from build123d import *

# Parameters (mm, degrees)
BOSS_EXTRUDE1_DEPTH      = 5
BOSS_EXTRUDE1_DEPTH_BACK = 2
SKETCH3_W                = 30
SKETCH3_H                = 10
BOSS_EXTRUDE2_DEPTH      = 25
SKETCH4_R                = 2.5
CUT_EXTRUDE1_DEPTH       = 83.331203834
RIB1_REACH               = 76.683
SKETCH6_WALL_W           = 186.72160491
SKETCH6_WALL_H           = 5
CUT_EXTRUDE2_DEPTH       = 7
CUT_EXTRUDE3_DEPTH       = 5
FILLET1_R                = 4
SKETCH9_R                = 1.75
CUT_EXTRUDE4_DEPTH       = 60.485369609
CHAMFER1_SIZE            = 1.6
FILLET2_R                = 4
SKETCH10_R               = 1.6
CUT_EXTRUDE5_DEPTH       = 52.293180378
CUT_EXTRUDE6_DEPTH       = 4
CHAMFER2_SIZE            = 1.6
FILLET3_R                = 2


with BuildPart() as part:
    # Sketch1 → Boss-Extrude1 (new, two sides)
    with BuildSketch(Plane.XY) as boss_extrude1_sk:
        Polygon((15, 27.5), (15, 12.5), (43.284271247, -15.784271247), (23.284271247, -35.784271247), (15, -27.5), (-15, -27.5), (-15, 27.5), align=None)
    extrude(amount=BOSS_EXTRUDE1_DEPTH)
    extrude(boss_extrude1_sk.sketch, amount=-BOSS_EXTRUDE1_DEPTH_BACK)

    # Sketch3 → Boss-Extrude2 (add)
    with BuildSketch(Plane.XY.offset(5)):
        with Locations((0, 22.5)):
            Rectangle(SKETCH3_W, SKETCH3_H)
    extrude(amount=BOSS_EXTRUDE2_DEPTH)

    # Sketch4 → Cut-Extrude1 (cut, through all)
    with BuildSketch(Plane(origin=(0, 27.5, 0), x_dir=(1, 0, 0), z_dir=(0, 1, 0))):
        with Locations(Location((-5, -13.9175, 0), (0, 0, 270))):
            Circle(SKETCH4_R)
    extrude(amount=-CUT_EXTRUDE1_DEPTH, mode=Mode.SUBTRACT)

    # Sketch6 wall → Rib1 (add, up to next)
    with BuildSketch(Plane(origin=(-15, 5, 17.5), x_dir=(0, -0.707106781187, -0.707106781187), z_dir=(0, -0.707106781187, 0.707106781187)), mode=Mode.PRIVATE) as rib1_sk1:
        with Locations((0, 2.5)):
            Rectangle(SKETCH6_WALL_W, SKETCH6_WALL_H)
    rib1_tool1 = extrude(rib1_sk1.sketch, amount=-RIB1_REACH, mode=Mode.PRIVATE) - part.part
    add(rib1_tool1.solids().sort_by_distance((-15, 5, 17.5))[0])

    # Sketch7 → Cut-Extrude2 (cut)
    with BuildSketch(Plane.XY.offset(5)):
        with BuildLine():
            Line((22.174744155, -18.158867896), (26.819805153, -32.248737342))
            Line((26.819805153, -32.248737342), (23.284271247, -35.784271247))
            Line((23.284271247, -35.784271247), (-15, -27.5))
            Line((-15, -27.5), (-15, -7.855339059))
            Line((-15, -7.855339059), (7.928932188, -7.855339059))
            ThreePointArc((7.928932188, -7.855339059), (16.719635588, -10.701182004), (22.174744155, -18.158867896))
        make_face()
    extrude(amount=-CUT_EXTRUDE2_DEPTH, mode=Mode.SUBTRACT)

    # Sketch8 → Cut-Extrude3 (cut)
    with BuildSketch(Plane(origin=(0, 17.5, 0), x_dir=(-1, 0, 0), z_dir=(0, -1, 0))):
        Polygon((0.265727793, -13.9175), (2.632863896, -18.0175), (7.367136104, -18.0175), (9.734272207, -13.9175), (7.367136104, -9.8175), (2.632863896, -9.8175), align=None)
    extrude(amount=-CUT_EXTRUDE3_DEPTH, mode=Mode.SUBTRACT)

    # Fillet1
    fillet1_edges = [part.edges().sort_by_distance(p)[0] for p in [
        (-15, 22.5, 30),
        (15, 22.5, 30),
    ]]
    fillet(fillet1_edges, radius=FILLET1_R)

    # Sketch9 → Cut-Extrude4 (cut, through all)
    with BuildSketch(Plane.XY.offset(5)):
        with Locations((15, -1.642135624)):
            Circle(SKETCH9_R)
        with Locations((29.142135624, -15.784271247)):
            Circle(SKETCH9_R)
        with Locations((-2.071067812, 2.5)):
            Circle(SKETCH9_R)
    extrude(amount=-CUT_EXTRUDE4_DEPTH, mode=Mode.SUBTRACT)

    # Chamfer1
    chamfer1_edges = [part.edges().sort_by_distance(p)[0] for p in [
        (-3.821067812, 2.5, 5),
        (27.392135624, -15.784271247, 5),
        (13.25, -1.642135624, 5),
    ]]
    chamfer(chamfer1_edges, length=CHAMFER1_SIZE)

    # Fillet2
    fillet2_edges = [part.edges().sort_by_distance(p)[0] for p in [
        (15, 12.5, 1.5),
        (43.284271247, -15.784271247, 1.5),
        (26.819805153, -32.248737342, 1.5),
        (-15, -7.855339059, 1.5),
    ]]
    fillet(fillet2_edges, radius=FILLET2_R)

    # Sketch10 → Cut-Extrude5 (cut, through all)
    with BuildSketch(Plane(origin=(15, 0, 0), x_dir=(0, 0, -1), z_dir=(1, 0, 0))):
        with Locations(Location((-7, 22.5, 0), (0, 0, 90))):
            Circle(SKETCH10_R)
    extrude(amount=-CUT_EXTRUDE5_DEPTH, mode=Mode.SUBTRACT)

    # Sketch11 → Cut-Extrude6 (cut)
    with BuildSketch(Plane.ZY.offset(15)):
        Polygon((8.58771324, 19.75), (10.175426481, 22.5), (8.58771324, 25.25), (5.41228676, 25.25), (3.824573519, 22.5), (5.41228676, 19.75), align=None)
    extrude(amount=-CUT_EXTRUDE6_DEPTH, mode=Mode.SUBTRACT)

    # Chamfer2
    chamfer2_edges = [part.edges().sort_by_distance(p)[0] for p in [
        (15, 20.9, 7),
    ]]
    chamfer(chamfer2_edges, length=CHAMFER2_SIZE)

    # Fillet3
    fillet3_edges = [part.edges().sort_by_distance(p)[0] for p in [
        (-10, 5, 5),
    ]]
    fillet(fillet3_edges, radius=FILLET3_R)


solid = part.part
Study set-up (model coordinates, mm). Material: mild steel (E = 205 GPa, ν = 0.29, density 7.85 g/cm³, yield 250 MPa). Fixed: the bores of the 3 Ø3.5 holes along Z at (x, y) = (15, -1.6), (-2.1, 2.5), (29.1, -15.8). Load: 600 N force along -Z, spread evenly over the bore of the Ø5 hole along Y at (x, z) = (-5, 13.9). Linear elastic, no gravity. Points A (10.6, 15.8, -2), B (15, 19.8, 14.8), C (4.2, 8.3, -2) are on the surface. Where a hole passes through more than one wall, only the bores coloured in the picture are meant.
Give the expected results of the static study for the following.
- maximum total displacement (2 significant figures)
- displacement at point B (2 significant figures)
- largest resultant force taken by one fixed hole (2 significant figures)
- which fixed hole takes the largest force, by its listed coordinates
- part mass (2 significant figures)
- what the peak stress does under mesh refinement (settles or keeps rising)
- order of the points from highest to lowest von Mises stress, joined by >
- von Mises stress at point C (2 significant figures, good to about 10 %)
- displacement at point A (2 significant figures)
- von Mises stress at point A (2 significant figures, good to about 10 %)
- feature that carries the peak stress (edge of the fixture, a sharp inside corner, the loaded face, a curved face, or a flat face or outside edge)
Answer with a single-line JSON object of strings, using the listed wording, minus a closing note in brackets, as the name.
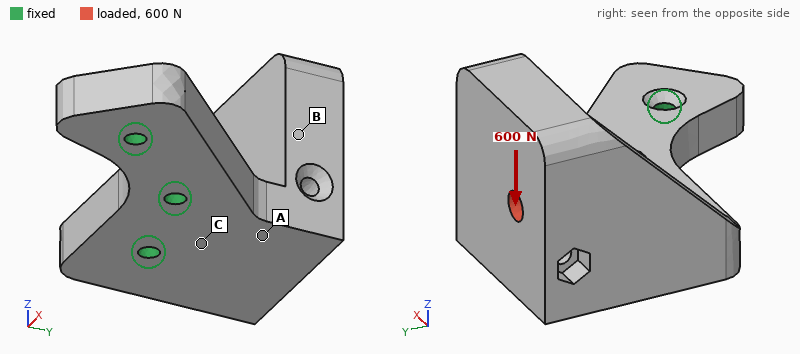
{"maximum total displacement": "30 µm", "displacement at point B": "14 µm", "largest resultant force taken by one fixed hole": "700 N", "which fixed hole takes the largest force, by its listed coordinates": "(-2.1, 2.5)", "part mass": "150 g", "what the peak stress does under mesh refinement": "keeps rising", "order of the points from highest to lowest von Mises stress, joined by >": "C > A > B", "von Mises stress at point C": "28 MPa", "displacement at point A": "7.1 µm", "von Mises stress at point A": "18 MPa", "feature that carries the peak stress": "edge of the fixture"}
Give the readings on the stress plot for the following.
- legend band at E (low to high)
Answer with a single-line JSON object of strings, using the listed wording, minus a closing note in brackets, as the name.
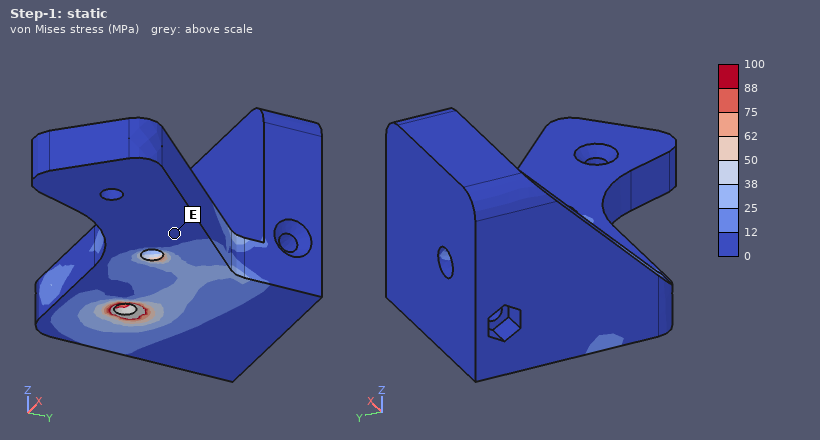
{"legend band at E": "0 to 12 MPa"}
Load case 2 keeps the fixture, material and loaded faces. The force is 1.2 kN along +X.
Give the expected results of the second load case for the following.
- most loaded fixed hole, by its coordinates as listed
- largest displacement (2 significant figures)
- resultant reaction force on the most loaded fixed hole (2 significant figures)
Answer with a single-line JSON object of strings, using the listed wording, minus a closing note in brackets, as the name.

{"most loaded fixed hole, by its coordinates as listed": "(-2.1, 2.5)", "largest displacement": "24 µm", "resultant reaction force on the most loaded fixed hole": "1.7 kN"}
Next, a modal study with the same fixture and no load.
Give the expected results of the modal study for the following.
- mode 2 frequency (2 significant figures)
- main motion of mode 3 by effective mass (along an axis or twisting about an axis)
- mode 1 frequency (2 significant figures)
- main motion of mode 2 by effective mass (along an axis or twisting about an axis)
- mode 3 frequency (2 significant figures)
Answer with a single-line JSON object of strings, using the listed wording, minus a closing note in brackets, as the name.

{"mode 2 frequency": "4500 Hz", "main motion of mode 3 by effective mass": "along Z", "mode 1 frequency": "3000 Hz", "main motion of mode 2 by effective mass": "along X", "mode 3 frequency": "11 kHz"}
